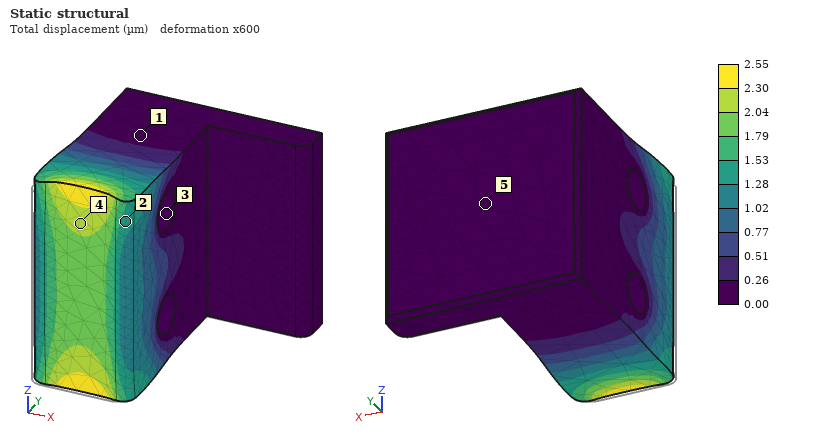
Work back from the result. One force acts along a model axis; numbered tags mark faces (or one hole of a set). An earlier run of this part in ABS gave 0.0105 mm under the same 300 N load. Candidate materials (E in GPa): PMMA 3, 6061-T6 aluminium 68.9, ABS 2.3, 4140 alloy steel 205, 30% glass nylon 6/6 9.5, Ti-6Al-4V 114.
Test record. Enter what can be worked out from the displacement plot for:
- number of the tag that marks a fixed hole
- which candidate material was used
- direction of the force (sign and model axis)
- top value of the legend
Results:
3
30% glass nylon 6/6
+Y
2.55 µm
